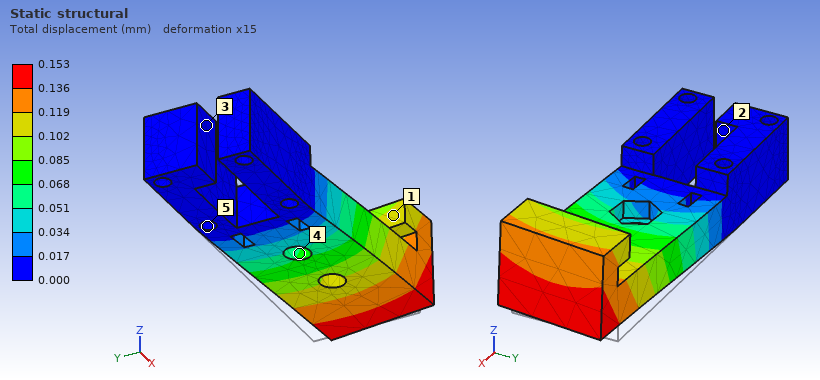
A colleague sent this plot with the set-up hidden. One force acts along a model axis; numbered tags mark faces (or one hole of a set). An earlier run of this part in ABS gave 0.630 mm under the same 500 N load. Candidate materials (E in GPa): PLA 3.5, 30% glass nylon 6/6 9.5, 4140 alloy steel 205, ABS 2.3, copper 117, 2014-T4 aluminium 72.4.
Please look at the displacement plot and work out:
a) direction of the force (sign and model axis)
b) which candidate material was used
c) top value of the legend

-Y
30% glass nylon 6/6
0.153 mm
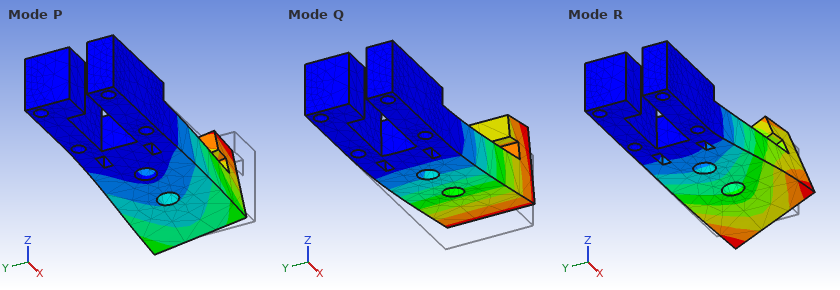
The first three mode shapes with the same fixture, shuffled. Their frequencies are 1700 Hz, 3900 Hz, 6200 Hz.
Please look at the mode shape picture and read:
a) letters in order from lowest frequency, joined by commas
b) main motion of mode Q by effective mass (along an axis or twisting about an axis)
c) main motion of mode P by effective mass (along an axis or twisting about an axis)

Q, P, R
along Z
along Y
